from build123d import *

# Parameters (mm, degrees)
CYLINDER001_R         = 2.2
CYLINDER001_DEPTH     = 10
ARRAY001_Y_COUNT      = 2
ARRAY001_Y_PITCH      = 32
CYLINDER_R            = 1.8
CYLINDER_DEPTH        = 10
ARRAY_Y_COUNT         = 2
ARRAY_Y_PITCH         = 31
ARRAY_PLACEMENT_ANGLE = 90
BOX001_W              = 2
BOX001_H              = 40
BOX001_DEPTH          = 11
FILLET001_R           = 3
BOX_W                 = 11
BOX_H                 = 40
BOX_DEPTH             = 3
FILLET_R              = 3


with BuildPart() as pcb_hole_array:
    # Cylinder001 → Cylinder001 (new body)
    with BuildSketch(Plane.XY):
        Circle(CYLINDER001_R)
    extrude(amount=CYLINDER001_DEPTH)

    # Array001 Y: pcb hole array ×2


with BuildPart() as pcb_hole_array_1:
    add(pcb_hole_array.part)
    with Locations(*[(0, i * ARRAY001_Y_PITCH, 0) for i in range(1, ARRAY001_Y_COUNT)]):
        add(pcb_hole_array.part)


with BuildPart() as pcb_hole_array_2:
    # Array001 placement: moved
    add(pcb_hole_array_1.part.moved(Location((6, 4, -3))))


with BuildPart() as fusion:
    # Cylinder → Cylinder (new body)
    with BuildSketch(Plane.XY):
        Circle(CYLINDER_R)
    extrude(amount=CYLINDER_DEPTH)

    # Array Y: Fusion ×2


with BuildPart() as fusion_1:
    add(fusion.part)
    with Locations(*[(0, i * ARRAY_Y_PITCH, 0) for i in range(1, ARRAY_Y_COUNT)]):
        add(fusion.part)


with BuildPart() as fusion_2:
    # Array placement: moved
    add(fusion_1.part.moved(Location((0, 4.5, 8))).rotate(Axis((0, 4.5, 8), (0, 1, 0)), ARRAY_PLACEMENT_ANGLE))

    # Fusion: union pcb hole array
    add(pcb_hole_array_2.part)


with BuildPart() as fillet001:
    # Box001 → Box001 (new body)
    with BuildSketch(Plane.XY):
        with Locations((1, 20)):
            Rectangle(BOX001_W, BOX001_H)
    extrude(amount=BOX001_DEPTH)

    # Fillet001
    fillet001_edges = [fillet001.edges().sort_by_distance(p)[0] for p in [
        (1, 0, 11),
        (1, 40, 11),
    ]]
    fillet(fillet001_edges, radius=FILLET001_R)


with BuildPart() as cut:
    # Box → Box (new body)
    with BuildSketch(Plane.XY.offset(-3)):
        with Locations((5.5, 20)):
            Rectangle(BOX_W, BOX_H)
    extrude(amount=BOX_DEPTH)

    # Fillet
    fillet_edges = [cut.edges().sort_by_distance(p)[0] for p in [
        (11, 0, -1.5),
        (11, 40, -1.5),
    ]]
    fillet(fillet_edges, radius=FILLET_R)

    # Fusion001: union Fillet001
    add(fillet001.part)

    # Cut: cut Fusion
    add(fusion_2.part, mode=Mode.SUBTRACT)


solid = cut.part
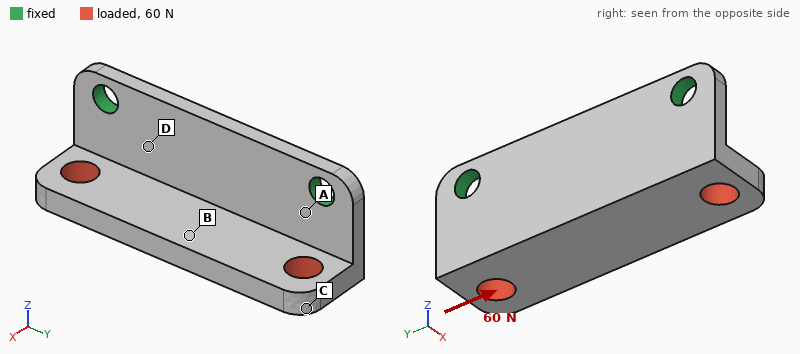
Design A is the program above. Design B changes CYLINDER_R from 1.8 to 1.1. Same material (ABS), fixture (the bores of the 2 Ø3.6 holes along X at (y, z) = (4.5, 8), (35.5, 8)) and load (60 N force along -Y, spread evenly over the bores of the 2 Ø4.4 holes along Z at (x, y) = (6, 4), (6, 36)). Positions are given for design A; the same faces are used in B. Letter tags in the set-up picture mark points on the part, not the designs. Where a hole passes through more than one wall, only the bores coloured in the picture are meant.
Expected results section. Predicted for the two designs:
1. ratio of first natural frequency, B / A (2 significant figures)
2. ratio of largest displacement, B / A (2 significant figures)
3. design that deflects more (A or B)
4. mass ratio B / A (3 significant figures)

0.87
1.2
B
1.01
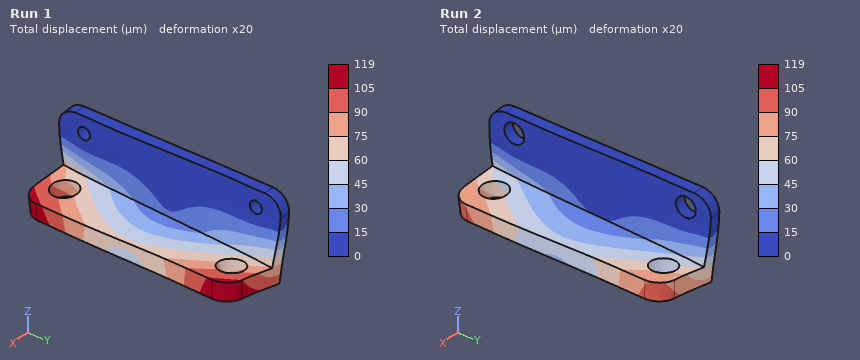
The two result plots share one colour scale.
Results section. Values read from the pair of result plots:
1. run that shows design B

Run 1
